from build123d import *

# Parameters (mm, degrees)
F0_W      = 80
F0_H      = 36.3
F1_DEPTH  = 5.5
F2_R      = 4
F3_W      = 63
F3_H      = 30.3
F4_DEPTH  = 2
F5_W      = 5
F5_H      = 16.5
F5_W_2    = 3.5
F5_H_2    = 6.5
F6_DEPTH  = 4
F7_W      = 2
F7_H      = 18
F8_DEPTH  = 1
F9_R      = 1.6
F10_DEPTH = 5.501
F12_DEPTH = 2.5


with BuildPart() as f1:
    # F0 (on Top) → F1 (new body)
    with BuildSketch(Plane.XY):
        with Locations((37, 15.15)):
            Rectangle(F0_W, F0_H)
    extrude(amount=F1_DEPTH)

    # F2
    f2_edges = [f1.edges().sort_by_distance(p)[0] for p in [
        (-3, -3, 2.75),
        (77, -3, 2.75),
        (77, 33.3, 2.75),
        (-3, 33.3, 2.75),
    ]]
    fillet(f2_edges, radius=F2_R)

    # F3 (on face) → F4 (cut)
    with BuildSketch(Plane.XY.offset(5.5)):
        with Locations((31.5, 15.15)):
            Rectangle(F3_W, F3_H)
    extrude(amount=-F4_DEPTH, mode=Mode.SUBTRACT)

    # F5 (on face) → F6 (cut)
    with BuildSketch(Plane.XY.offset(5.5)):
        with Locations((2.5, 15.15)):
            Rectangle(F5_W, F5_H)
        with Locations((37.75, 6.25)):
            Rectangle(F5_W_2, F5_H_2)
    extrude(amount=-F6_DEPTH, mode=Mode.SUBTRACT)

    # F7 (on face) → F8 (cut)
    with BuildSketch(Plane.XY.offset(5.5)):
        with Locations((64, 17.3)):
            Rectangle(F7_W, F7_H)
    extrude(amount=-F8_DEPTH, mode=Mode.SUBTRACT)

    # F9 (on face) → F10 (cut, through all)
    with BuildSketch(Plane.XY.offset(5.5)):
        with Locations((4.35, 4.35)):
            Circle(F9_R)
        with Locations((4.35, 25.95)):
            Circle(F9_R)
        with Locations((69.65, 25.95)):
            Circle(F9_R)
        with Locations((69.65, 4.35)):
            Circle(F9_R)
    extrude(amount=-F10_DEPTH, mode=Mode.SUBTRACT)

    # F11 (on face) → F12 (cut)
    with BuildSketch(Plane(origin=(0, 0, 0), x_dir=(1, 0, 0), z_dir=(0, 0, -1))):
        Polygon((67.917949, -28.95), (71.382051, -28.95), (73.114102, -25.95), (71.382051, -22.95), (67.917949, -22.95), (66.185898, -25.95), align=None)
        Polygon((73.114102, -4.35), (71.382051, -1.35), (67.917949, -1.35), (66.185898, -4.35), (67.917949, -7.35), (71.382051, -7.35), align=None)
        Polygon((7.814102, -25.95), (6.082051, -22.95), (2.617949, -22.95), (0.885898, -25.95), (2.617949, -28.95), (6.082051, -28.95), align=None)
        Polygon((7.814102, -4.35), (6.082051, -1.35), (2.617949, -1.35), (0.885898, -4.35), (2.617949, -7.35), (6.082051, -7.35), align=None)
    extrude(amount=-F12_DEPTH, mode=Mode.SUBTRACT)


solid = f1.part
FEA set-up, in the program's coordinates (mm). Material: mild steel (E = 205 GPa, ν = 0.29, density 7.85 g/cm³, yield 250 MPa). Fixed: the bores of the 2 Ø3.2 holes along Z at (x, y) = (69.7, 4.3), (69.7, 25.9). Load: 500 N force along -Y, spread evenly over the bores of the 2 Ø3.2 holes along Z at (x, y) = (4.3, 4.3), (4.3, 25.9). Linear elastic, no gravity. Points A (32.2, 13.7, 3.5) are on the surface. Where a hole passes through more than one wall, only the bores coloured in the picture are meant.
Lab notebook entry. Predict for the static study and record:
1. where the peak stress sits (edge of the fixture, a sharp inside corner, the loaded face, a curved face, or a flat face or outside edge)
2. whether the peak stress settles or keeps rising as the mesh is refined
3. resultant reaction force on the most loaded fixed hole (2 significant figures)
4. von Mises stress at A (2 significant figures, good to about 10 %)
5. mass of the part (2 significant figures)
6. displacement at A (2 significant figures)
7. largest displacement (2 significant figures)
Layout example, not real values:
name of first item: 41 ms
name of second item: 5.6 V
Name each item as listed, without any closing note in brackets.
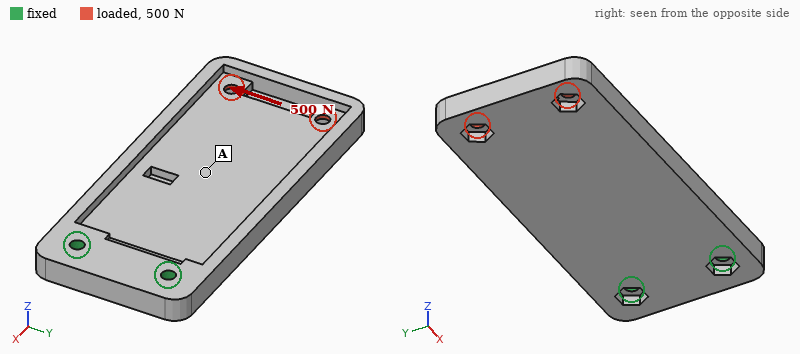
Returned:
where the peak stress sits: edge of the fixture
whether the peak stress settles or keeps rising as the mesh is refined: keeps rising
resultant reaction force on the most loaded fixed hole: 1.4 kN
von Mises stress at A: 18 MPa
mass of the part: 90 g
displacement at A: 13 µm
largest displacement: 43 µm
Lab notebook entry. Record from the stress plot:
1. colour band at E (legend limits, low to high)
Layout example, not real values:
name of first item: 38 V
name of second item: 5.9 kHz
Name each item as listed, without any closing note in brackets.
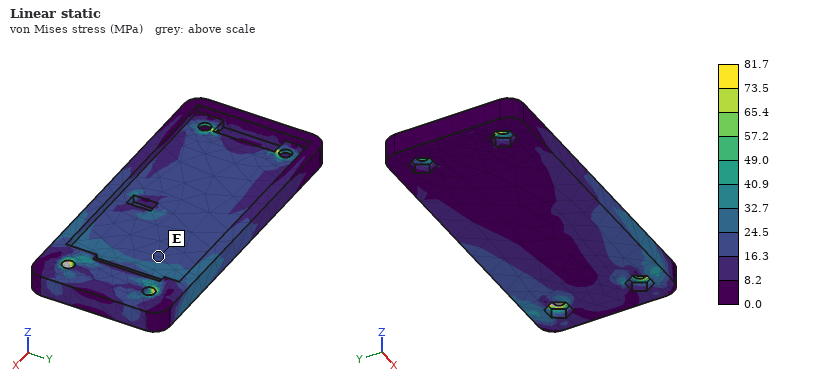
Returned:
colour band at E: 16.3 to 24.5 MPa
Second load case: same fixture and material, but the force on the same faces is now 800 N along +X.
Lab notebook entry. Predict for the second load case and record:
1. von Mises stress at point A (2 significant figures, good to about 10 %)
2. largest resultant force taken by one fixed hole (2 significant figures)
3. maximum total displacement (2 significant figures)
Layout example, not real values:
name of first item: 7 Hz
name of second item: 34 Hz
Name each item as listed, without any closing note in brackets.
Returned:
von Mises stress at point A: 12 MPa
largest resultant force taken by one fixed hole: 400 N
maximum total displacement: 37 µm
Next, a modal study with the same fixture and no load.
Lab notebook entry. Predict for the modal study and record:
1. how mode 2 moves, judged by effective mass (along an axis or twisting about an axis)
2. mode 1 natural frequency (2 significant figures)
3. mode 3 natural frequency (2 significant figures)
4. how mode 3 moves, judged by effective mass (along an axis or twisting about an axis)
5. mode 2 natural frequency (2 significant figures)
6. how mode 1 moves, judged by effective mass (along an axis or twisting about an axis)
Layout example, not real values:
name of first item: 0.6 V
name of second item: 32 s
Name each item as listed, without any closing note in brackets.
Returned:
how mode 2 moves, judged by effective mass: twisting about X
mode 1 natural frequency: 660 Hz
mode 3 natural frequency: 3900 Hz
how mode 3 moves, judged by effective mass: along Z
mode 2 natural frequency: 2300 Hz
how mode 1 moves, judged by effective mass: along Z
